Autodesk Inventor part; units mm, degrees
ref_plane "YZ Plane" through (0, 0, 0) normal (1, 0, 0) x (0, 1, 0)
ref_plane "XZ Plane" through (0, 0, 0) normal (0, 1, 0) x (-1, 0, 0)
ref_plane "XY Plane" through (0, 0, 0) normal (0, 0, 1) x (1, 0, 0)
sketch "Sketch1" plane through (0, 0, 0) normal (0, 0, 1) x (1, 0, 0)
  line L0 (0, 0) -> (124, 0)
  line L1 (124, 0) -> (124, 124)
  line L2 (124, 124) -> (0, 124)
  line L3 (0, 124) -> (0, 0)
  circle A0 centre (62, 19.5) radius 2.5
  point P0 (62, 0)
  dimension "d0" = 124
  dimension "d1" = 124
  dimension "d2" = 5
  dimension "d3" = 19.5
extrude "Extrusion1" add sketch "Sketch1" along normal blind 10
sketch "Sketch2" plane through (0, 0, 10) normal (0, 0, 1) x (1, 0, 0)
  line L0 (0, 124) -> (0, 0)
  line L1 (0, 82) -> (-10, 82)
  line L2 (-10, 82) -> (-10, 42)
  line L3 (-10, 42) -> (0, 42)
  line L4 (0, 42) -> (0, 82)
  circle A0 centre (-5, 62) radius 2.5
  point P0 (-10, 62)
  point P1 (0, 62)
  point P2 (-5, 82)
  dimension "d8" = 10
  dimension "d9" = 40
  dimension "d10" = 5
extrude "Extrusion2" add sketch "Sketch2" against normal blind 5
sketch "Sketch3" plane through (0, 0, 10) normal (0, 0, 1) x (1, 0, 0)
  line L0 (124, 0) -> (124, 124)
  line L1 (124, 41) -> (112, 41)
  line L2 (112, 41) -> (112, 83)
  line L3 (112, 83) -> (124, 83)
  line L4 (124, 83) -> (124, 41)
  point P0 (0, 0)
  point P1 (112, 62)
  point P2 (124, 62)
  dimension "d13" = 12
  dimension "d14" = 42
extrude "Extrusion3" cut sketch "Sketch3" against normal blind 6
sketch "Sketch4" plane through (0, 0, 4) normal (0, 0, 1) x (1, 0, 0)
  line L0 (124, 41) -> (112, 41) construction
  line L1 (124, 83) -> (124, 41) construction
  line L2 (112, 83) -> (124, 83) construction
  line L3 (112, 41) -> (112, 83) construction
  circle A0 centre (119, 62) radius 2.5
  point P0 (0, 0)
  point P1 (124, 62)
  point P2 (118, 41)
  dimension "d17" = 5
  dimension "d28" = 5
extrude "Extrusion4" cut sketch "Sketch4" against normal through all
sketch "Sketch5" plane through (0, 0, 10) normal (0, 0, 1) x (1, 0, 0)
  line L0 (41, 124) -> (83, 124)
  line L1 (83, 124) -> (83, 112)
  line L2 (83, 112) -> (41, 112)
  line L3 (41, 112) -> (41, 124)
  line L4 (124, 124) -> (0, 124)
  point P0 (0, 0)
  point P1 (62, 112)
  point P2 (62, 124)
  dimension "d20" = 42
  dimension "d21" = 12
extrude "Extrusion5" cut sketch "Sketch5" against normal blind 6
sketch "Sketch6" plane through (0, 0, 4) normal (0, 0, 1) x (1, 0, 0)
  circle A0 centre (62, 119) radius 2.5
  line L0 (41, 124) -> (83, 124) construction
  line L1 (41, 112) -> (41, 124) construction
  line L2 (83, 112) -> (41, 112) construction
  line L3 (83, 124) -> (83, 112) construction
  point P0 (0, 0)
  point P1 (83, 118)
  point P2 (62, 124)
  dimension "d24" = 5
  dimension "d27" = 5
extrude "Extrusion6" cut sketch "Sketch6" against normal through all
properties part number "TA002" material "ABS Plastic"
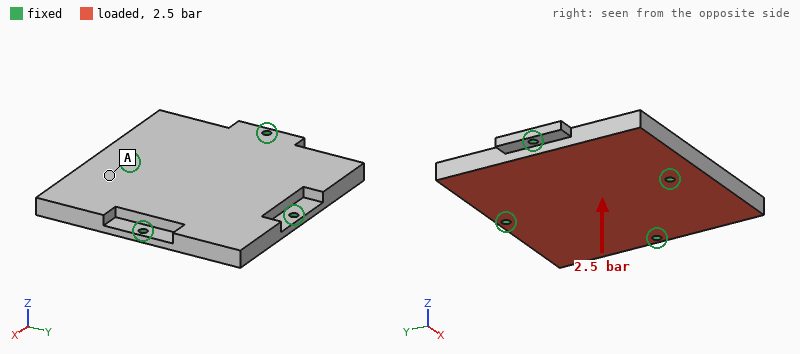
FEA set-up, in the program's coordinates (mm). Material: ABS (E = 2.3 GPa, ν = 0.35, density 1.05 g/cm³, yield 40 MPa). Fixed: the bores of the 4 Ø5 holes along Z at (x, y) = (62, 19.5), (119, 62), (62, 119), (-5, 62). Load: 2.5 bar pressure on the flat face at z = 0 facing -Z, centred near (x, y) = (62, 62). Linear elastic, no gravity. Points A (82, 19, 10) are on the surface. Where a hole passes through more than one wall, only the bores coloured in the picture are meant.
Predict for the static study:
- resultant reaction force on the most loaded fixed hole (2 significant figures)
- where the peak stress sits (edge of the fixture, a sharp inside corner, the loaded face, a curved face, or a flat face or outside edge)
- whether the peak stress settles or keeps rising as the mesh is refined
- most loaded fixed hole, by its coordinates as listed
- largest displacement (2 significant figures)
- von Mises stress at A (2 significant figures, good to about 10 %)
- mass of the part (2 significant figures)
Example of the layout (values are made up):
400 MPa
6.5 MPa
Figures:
1.4 kN
edge of the fixture
keeps rising
(62, 19.5)
1.4 mm
4.8 MPa
160 g
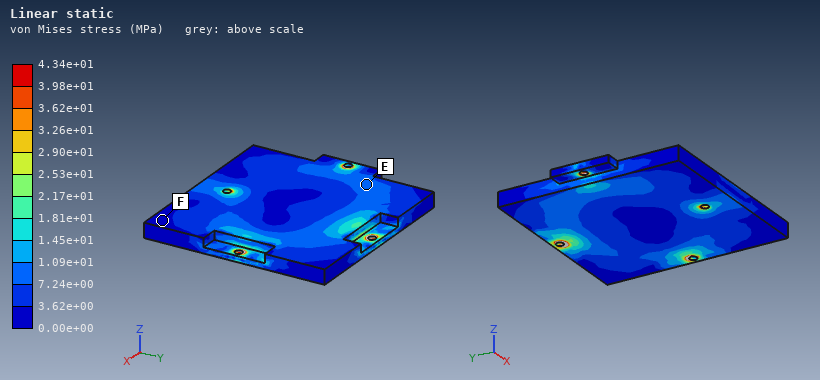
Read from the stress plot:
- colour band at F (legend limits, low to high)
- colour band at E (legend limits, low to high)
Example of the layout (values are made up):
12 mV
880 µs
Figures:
0.00e+00 to 3.62e+00 MPa
7.24e+00 to 1.09e+01 MPa
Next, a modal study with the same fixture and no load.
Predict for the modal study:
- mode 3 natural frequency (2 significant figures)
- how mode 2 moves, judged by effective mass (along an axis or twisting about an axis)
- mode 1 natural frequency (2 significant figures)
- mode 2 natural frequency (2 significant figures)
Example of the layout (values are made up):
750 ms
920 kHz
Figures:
910 Hz
along Z
740 Hz
840 Hz
